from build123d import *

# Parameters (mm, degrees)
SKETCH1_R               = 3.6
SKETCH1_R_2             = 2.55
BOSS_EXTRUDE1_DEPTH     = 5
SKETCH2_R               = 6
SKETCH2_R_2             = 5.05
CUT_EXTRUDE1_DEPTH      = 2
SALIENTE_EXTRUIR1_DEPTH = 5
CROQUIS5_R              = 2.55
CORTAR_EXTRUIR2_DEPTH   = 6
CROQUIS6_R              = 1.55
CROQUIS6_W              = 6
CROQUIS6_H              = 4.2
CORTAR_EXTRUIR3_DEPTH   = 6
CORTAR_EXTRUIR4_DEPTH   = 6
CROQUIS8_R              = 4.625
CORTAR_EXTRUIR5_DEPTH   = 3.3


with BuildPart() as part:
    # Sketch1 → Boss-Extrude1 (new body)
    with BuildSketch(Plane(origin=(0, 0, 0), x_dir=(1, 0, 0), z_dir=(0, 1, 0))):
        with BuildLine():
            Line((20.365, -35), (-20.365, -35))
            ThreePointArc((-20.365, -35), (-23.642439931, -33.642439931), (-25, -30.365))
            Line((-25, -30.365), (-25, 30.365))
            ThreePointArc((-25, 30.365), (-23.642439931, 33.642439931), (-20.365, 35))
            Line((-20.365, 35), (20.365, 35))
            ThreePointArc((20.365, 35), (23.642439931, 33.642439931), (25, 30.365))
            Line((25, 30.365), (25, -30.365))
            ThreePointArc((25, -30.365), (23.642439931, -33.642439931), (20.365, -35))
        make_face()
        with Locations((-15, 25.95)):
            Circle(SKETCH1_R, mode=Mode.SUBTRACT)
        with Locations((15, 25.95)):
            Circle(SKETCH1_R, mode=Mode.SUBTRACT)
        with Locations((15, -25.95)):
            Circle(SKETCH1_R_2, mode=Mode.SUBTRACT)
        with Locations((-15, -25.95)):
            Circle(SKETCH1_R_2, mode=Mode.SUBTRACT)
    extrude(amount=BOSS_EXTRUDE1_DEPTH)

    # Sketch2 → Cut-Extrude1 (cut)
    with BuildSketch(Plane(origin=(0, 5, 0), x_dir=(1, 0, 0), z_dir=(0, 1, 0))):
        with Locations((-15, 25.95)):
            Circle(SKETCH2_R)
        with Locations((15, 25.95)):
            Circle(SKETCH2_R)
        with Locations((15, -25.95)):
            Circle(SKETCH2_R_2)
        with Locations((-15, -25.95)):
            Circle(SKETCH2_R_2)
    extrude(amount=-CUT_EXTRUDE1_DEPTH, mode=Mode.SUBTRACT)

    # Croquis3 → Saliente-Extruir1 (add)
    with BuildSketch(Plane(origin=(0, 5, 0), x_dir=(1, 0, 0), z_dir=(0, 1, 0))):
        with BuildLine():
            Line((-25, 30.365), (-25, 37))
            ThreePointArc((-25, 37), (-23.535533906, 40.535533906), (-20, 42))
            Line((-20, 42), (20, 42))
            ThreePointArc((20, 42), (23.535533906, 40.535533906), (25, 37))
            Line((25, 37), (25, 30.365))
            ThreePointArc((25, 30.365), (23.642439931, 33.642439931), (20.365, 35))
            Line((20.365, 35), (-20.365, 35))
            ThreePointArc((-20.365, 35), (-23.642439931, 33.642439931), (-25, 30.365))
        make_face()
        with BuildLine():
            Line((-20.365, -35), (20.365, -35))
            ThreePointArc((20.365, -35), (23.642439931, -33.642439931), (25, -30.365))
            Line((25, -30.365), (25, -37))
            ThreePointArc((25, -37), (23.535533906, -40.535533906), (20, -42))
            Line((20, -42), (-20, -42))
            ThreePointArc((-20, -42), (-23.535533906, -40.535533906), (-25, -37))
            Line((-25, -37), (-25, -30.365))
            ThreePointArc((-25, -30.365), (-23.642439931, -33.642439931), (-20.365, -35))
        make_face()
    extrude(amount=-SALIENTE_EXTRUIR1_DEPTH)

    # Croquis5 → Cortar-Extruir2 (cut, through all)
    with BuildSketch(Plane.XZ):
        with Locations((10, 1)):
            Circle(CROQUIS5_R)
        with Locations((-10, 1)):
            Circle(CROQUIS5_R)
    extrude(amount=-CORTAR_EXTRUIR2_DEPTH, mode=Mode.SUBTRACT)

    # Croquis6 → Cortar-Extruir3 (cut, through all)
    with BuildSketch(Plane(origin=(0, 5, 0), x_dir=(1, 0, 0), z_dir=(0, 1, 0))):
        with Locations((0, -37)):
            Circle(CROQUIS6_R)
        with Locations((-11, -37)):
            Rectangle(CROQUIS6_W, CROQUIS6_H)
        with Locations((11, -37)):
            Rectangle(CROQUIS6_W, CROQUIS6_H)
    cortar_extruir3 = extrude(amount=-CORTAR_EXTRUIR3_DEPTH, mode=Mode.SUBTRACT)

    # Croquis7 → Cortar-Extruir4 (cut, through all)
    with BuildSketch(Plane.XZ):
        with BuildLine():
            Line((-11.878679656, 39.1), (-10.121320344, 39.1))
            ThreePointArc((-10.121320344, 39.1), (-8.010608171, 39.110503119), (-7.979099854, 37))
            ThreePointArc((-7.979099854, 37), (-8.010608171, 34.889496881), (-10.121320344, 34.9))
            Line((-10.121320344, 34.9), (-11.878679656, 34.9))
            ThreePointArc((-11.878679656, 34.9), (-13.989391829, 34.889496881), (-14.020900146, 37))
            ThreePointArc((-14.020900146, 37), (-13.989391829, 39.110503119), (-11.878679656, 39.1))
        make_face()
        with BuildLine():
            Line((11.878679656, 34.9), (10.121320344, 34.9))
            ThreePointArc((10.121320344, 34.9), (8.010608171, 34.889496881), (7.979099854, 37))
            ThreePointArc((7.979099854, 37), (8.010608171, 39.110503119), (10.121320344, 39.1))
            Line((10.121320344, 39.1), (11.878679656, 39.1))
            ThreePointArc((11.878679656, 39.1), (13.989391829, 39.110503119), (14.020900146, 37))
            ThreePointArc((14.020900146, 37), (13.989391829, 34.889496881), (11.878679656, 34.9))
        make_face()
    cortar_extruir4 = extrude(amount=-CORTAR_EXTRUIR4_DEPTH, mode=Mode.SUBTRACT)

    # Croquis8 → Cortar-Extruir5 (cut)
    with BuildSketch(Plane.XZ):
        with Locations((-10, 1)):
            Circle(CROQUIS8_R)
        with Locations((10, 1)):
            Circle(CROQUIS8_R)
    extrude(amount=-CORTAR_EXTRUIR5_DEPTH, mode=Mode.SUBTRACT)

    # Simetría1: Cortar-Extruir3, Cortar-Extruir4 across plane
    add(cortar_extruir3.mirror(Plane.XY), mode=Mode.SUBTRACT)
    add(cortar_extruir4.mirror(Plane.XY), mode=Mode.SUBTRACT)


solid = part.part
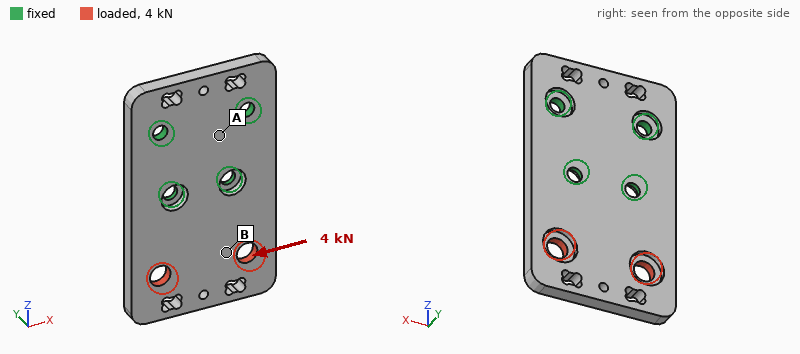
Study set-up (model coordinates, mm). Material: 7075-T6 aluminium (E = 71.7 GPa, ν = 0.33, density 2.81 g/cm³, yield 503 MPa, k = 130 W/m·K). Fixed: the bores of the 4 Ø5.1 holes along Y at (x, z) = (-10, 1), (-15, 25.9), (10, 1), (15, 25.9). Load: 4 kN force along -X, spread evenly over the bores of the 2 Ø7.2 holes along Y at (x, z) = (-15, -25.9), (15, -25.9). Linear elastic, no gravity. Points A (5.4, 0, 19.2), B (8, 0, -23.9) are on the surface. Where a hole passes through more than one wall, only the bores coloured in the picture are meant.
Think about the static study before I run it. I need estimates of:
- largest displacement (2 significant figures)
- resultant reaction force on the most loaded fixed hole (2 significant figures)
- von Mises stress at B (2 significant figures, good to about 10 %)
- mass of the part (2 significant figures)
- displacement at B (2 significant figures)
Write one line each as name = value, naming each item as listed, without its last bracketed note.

largest displacement = 81 µm
resultant reaction force on the most loaded fixed hole = 3.2 kN
von Mises stress at B = 48 MPa
mass of the part = 52 g
displacement at B = 45 µm
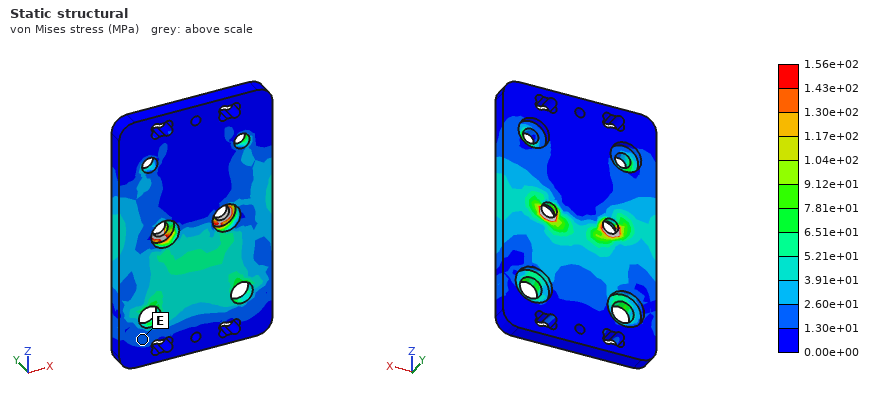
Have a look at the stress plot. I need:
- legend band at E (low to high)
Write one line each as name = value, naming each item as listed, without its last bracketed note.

legend band at E = 1.30e+01 to 2.60e+01 MPa
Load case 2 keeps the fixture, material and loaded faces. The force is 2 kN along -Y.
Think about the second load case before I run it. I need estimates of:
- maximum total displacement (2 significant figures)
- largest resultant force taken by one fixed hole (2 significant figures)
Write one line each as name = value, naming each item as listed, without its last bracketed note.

maximum total displacement = 1.00 mm
largest resultant force taken by one fixed hole = 2.6 kN
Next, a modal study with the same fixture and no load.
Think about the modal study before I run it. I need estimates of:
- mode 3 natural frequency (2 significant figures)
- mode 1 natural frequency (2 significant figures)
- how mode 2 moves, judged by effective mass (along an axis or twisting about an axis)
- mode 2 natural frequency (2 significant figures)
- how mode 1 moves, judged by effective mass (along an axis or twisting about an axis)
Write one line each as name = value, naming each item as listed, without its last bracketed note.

mode 3 natural frequency = 9300 Hz
mode 1 natural frequency = 2000 Hz
how mode 2 moves, judged by effective mass = twisting about Z
mode 2 natural frequency = 3900 Hz
how mode 1 moves, judged by effective mass = along Y
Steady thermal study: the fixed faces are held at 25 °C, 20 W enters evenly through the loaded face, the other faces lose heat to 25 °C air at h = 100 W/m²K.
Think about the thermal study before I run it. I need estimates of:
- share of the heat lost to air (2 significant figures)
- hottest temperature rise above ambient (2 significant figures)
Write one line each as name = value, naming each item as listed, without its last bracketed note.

share of the heat lost to air = 33 %
hottest temperature rise above ambient = 20 K
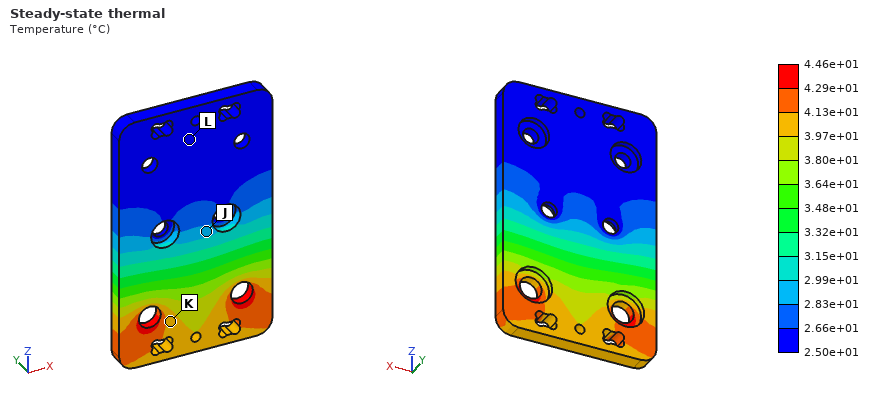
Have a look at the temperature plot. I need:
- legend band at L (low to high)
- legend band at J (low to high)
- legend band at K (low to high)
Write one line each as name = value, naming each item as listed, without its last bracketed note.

legend band at L = 2.50e+01 to 2.66e+01 °C
legend band at J = 2.83e+01 to 2.99e+01 °C
legend band at K = 3.97e+01 to 4.13e+01 °C
